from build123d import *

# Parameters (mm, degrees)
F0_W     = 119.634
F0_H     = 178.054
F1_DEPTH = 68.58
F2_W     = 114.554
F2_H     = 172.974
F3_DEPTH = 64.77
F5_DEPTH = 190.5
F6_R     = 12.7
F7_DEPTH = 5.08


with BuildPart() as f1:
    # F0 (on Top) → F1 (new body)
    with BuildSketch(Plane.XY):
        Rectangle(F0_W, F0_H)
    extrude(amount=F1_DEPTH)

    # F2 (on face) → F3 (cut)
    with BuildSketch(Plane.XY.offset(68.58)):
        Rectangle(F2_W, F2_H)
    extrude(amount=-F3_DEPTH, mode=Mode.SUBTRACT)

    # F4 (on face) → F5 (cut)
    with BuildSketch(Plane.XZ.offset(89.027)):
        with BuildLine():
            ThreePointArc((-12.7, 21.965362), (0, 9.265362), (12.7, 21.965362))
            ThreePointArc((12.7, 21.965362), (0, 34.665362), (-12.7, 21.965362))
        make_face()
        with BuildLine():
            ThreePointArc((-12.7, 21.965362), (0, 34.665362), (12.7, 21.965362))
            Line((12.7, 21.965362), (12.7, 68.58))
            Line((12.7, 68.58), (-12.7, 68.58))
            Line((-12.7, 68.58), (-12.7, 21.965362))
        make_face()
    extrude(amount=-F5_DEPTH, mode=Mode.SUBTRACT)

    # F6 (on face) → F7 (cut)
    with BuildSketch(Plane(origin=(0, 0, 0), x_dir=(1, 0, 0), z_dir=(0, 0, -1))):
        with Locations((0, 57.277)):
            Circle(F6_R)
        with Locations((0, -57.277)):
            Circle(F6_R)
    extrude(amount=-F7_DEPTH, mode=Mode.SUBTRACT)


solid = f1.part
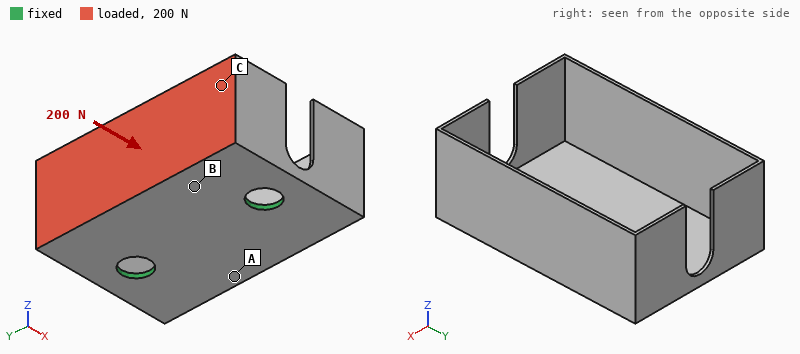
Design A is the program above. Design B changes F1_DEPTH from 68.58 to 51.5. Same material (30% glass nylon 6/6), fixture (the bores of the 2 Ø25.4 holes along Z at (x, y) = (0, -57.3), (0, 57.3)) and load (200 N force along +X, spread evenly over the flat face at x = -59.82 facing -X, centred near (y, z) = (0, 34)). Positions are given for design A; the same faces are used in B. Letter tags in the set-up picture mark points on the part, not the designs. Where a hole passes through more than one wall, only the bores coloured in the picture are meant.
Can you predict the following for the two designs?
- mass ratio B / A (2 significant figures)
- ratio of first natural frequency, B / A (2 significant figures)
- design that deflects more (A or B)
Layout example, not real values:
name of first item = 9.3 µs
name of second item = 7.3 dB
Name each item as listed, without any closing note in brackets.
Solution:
mass ratio B / A = 0.86
ratio of first natural frequency, B / A = 1.3
design that deflects more = A
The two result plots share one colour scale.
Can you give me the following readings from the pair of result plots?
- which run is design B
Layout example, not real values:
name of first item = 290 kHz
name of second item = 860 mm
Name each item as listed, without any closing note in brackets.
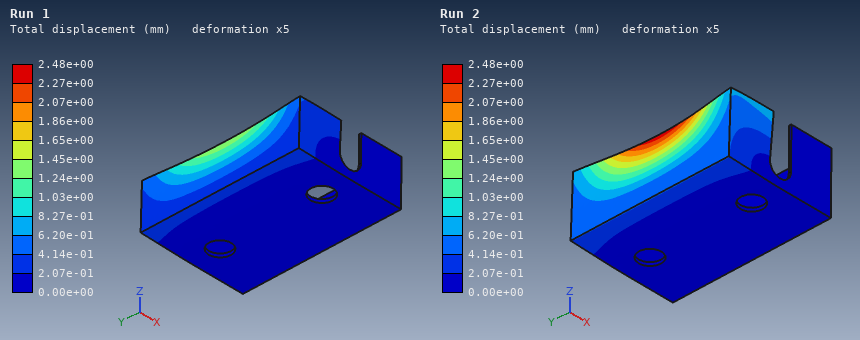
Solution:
which run is design B = Run 1
